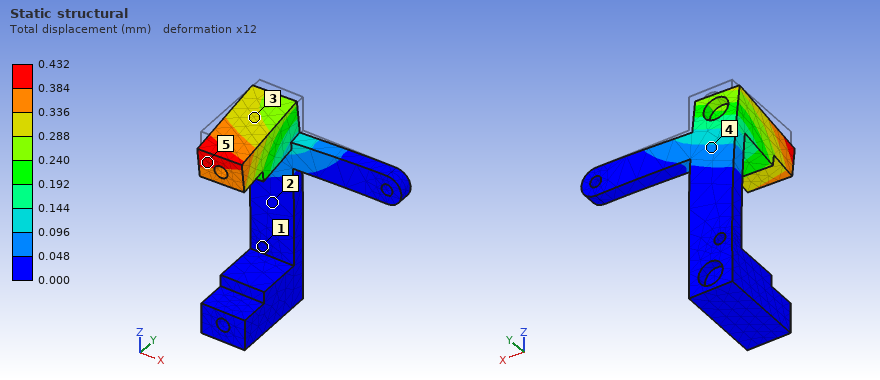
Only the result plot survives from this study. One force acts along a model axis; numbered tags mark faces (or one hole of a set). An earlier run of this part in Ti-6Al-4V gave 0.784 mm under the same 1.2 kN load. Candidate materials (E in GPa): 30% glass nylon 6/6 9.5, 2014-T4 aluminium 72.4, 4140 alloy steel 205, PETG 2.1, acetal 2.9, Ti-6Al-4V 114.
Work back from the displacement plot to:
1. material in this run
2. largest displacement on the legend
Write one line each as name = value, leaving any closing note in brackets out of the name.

material in this run = 4140 alloy steel
largest displacement on the legend = 0.432 mm
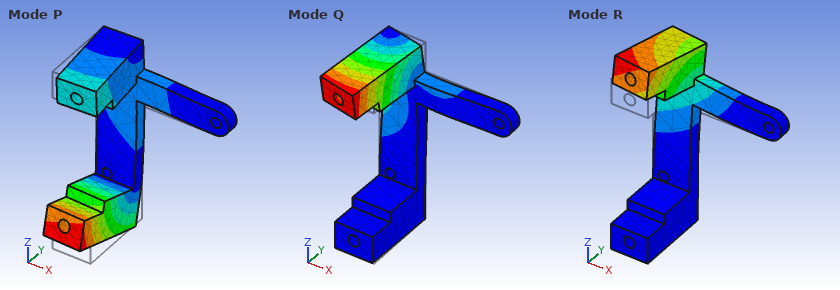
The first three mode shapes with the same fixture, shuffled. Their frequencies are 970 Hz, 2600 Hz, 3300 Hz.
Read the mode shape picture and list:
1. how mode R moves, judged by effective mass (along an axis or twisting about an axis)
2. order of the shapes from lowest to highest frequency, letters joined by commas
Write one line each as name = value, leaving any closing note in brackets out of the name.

how mode R moves, judged by effective mass = along Y
order of the shapes from lowest to highest frequency, letters joined by commas = R, Q, P
